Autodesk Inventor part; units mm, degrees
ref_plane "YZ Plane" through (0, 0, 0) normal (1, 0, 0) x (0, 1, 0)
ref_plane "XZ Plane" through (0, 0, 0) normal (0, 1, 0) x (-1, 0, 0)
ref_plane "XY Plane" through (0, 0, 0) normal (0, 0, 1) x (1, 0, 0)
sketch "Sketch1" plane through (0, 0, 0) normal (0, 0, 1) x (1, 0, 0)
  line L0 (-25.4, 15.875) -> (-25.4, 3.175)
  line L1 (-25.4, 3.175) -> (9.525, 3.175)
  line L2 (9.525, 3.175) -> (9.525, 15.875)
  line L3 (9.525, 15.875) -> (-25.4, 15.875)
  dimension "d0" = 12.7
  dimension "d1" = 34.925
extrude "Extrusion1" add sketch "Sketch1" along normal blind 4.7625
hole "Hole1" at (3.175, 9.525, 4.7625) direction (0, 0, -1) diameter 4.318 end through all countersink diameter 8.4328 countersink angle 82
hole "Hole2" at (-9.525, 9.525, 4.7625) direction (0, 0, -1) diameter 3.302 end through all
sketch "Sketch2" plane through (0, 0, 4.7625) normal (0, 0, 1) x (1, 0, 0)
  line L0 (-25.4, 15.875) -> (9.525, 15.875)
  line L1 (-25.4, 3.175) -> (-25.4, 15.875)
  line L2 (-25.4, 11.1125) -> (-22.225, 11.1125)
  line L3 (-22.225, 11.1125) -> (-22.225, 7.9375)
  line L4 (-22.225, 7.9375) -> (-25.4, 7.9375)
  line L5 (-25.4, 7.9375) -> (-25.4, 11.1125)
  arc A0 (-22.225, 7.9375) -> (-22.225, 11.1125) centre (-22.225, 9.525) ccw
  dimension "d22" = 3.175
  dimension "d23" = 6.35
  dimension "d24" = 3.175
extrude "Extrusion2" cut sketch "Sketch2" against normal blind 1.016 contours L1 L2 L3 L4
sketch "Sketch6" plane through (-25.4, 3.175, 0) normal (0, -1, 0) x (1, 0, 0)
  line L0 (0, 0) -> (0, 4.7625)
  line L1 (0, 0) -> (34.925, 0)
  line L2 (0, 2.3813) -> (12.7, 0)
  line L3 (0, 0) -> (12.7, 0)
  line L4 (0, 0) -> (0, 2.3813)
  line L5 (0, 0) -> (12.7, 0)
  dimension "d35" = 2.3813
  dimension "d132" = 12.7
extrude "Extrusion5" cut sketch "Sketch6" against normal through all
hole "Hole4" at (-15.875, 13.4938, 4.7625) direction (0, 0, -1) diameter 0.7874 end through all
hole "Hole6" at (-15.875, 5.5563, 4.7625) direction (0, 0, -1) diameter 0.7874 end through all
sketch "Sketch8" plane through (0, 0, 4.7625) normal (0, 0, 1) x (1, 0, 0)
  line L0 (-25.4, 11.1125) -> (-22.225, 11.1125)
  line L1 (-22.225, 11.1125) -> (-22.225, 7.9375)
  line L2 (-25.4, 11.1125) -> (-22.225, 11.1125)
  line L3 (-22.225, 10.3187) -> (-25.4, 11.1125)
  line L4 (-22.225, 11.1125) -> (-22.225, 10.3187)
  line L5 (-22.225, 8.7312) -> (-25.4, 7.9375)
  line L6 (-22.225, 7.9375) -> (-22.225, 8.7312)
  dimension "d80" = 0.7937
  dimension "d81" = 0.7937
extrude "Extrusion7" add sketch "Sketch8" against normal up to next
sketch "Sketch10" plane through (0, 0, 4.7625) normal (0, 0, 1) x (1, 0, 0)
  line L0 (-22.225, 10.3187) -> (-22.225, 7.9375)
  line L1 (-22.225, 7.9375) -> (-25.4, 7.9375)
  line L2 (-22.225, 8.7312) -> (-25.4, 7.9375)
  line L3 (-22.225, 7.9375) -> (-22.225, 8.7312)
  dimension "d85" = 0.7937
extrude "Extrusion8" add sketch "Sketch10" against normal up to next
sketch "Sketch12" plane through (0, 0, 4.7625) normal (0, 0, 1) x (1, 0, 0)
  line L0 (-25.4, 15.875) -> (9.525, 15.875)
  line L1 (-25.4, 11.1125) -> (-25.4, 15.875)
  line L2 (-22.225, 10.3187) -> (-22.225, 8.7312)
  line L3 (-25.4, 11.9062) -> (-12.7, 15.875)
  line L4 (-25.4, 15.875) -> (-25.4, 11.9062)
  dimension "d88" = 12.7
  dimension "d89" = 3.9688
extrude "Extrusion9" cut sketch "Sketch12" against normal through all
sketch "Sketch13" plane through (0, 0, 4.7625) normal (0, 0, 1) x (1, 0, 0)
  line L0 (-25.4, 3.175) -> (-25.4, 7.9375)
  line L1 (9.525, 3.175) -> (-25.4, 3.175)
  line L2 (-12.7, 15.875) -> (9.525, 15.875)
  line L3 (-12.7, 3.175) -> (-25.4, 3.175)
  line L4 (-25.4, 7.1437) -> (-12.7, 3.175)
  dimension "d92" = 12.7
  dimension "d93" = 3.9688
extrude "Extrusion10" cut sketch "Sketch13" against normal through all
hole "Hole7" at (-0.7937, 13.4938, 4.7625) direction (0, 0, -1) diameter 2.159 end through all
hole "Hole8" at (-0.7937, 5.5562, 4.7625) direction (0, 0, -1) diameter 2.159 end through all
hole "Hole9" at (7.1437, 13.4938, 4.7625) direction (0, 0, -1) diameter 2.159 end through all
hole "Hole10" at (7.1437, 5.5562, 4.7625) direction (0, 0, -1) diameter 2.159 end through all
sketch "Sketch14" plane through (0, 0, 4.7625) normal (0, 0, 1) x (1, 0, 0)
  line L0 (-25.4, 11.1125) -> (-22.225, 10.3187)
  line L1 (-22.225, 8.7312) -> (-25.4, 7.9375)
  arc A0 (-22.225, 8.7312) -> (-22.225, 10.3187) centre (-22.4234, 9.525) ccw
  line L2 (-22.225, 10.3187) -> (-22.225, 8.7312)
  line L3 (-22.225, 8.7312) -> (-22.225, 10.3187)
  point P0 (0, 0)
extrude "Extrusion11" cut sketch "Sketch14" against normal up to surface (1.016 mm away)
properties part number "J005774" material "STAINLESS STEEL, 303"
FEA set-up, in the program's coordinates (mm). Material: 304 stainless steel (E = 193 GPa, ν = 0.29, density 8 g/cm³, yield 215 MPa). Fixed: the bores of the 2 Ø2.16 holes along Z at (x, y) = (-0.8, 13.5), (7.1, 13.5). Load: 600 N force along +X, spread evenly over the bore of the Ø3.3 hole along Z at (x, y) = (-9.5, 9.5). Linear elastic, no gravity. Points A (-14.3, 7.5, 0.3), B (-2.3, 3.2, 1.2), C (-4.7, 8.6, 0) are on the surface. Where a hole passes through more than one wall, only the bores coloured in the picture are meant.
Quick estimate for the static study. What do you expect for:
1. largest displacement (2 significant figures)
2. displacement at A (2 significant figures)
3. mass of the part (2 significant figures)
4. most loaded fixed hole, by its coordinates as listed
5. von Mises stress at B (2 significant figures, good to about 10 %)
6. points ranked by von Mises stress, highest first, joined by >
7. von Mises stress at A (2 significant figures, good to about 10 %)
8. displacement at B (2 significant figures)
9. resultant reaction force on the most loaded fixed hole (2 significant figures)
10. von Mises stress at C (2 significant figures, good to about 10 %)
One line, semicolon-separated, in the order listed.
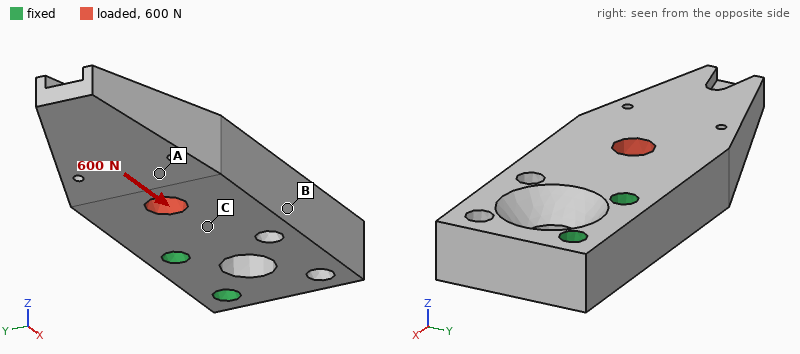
5.7 µm; 3.5 µm; 12 g; (-0.8, 13.5); 20 MPa; B > C > A; 5.6 MPa; 2.3 µm; 500 N; 11 MPa
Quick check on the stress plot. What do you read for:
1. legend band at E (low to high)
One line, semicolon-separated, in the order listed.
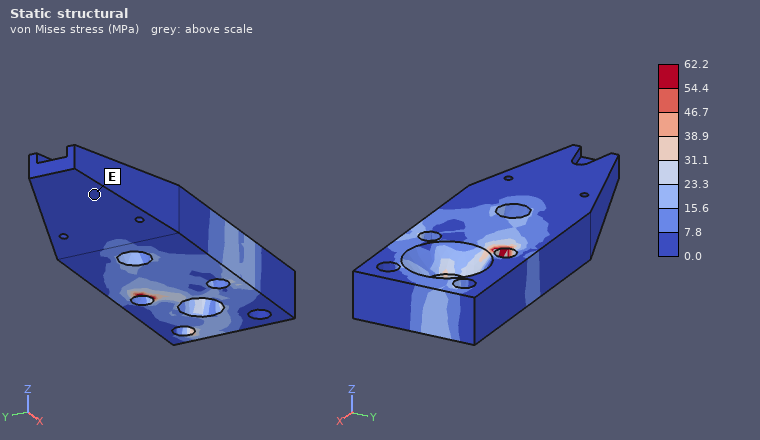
0.0 to 7.8 MPa
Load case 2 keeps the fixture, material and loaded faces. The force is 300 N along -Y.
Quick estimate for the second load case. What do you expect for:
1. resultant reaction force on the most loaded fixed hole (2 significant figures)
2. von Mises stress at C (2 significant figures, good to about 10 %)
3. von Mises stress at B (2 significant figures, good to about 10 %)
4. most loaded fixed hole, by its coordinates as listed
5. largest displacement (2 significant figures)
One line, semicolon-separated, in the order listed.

480 N; 11 MPa; 24 MPa; (-0.8, 13.5); 7.8 µm
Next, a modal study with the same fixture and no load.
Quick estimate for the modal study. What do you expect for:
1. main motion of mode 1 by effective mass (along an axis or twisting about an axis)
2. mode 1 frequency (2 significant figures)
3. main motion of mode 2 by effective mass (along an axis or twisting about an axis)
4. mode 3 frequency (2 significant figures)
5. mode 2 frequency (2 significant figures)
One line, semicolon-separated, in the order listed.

along Z; 7500 Hz; along Y; 20 kHz; 12 kHz
